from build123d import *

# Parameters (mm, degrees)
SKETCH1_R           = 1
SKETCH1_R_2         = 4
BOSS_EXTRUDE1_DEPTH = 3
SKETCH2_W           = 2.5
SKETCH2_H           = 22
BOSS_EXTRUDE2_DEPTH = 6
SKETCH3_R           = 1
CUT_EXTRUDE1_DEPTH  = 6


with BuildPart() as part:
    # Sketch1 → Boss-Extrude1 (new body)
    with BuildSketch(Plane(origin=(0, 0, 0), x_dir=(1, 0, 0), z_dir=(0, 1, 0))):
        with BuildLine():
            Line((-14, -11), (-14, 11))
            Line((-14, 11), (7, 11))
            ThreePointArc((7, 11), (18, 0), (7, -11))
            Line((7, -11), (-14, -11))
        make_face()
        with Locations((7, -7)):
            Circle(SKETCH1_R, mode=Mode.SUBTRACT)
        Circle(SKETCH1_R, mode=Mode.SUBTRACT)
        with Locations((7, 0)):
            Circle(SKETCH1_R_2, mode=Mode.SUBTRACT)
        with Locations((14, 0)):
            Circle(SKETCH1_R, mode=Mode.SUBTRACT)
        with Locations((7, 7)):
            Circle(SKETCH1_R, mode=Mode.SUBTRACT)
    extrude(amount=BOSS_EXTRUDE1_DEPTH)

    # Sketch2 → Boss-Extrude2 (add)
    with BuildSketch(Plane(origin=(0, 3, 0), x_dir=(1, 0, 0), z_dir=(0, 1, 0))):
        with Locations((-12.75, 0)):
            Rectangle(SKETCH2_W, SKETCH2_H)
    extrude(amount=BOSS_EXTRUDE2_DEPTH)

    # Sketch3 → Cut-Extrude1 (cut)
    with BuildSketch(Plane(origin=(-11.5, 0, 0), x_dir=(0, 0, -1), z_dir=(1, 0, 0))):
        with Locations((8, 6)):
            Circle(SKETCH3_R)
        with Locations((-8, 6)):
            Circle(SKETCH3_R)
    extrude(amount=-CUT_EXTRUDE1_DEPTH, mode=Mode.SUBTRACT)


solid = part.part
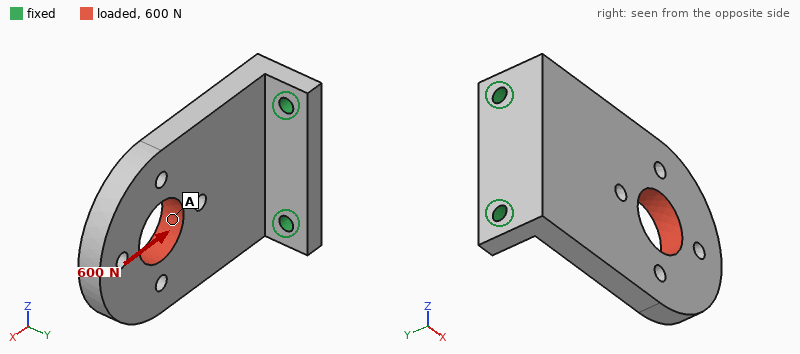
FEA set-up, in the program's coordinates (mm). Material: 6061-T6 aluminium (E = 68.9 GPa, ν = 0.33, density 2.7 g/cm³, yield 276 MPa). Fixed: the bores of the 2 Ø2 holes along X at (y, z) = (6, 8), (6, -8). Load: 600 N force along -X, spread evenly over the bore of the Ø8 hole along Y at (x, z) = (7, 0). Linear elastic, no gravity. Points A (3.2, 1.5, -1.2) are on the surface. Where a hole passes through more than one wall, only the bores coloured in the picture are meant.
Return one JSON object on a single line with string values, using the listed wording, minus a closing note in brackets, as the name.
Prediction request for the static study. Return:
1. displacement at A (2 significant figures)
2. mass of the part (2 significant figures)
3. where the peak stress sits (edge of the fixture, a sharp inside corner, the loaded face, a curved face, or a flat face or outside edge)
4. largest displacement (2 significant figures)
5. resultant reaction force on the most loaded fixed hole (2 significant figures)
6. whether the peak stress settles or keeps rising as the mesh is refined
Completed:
{"displacement at A": "0.064 mm", "mass of the part": "5.6 g", "where the peak stress sits": "edge of the fixture", "largest displacement": "0.12 mm", "resultant reaction force on the most loaded fixed hole": "300 N", "whether the peak stress settles or keeps rising as the mesh is refined": "keeps rising"}
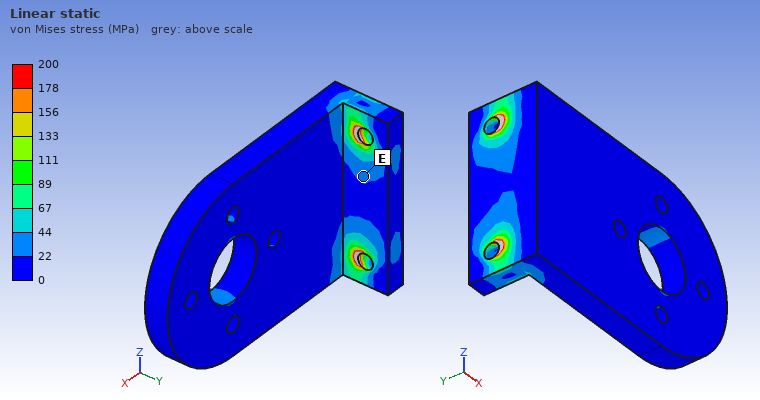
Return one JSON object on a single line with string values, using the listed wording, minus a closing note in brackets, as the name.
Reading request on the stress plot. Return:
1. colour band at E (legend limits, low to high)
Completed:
{"colour band at E": "22 to 44 MPa"}
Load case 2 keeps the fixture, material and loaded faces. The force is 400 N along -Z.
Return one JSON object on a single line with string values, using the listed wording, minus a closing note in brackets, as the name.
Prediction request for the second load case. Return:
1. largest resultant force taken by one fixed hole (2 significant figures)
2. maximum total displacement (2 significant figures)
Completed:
{"largest resultant force taken by one fixed hole": "520 N", "maximum total displacement": "70 µm"}
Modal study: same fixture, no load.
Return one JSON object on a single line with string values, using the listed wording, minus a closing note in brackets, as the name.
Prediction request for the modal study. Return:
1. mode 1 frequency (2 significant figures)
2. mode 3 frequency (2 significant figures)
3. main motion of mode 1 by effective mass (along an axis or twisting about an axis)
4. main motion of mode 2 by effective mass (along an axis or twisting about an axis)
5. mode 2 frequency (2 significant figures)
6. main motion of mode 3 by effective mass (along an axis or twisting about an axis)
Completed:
{"mode 1 frequency": "2200 Hz", "mode 3 frequency": "9700 Hz", "main motion of mode 1 by effective mass": "along Y", "main motion of mode 2 by effective mass": "along Z", "mode 2 frequency": "7300 Hz", "main motion of mode 3 by effective mass": "along Z"}
